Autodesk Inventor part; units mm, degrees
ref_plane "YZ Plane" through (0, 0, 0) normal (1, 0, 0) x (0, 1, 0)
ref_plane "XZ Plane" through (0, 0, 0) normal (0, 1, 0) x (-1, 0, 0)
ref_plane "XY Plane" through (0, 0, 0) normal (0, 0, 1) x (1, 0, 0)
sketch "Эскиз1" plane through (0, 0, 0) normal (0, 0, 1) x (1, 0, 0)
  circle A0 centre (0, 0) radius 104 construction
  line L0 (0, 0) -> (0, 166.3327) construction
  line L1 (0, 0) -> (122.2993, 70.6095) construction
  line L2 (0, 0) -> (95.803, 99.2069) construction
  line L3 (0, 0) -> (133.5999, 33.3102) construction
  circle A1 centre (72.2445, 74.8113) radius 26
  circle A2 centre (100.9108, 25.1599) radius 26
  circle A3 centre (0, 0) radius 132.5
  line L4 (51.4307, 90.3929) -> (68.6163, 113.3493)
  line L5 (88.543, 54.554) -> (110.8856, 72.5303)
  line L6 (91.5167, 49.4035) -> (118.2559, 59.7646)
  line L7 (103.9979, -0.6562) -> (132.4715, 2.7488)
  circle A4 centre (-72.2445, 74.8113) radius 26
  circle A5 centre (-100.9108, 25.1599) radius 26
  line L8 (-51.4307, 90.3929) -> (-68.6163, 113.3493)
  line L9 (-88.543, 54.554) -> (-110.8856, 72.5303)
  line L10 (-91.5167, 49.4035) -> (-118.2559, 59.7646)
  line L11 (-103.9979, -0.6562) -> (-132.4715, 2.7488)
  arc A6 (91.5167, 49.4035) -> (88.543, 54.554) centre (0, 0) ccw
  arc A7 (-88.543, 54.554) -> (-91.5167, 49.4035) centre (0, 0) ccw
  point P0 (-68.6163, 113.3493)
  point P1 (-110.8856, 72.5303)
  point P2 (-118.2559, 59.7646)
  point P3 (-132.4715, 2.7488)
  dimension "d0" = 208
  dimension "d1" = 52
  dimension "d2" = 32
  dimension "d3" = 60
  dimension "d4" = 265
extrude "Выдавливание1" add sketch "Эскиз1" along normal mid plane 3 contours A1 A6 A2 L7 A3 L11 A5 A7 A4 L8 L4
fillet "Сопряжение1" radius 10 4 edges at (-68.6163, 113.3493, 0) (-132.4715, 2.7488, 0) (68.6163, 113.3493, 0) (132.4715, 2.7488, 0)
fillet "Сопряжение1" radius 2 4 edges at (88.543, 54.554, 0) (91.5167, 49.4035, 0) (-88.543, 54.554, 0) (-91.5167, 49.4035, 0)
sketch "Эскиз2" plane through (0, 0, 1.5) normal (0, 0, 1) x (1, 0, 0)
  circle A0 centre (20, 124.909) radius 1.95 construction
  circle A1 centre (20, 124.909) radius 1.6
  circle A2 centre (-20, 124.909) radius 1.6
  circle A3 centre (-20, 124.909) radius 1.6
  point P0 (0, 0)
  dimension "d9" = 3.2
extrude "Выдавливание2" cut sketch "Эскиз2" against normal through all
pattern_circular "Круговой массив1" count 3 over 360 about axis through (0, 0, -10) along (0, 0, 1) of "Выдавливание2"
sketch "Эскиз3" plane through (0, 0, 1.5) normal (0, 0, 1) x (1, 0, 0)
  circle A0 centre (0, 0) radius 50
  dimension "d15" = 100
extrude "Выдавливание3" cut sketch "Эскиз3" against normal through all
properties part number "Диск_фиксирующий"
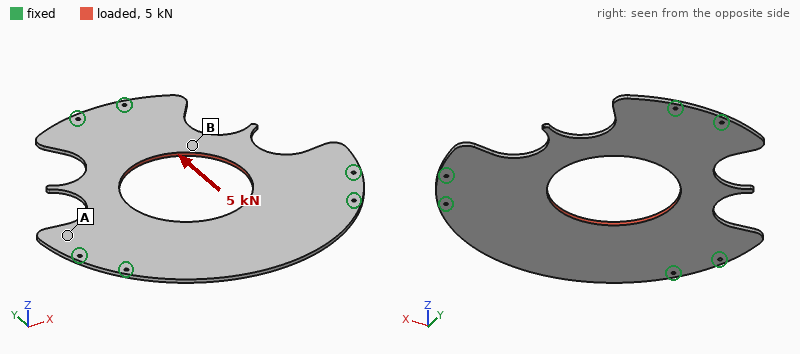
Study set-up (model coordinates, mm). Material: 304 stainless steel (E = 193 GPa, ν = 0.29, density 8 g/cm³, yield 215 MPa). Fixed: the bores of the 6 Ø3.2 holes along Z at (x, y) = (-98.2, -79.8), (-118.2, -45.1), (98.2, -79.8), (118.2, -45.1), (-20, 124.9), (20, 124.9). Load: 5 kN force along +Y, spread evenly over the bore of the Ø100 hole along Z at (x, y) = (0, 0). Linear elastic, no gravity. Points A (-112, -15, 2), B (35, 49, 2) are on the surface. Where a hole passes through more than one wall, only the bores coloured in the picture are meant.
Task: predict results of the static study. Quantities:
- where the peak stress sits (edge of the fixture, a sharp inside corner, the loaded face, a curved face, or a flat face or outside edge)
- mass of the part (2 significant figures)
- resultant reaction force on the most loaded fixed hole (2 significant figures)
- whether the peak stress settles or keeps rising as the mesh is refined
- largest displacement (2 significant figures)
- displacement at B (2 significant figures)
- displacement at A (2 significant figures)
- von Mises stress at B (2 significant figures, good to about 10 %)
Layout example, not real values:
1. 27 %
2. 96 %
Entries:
1. edge of the fixture
2. 870 g
3. 1.3 kN
4. keeps rising
5. 12 µm
6. 5.0 µm
7. 4.5 µm
8. 12 MPa
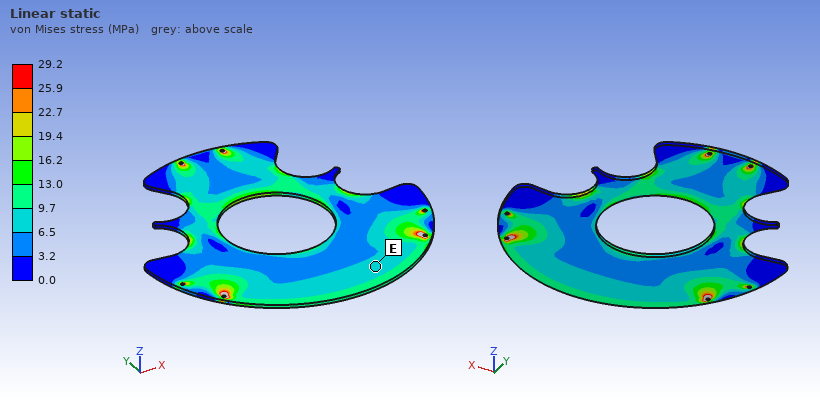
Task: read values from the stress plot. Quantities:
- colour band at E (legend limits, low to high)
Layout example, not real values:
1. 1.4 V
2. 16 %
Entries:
1. 6.5 to 9.7 MPa
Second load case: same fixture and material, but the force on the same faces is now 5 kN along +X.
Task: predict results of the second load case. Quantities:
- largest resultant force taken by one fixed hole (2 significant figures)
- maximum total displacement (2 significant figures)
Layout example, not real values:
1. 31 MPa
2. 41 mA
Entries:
1. 1.4 kN
2. 18 µm
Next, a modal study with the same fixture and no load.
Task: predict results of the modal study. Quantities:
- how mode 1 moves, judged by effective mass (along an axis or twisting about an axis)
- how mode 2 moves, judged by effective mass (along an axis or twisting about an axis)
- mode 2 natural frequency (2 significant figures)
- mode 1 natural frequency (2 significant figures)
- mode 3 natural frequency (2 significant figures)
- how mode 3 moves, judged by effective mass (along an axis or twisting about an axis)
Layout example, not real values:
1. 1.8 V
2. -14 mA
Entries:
1. along Z
2. along Z
3. 350 Hz
4. 310 Hz
5. 480 Hz
6. twisting about Y
